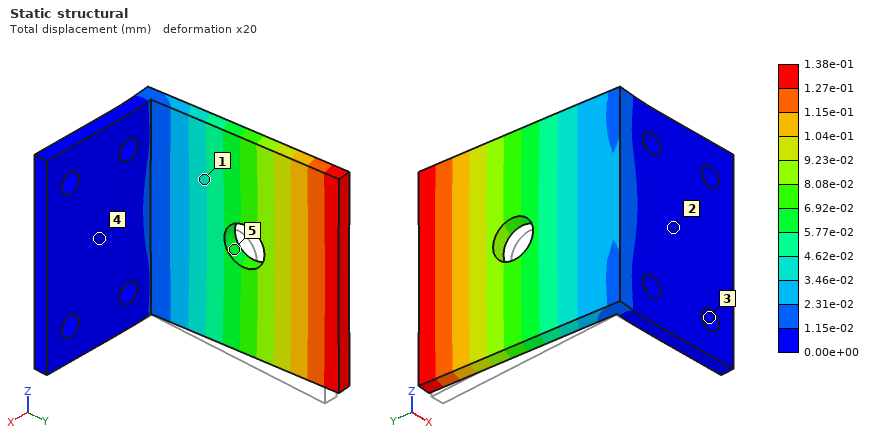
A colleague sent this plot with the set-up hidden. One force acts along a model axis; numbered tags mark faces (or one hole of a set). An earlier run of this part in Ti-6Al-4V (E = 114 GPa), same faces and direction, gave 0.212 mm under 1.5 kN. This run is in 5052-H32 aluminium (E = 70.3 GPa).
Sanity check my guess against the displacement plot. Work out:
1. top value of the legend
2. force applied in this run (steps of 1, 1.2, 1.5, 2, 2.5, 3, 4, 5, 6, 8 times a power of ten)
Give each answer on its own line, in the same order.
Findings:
1.38e-01 mm
600 N
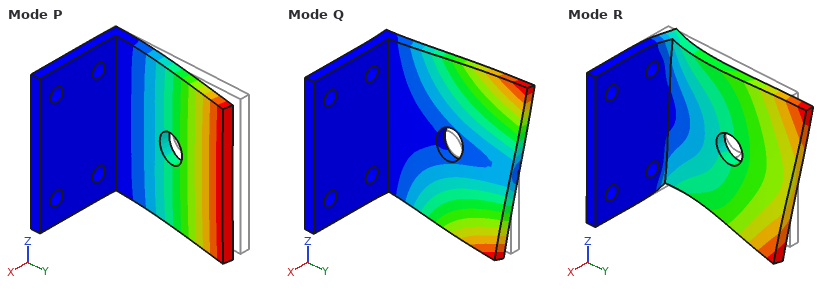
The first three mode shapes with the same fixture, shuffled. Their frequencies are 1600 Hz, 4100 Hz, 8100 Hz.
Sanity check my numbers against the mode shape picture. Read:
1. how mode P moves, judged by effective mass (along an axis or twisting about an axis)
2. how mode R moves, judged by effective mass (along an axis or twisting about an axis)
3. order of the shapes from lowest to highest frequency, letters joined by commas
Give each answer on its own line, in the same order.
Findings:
along X
along Z
P, Q, R
